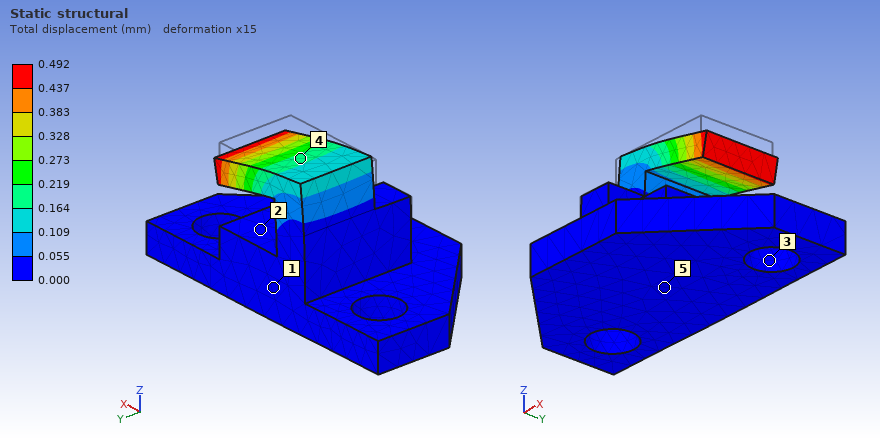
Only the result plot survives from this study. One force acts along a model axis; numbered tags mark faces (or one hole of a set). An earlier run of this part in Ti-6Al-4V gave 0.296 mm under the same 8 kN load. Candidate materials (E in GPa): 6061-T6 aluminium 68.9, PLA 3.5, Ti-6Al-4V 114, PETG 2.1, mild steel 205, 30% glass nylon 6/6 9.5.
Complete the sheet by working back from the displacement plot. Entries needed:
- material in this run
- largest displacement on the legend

6061-T6 aluminium
0.492 mm
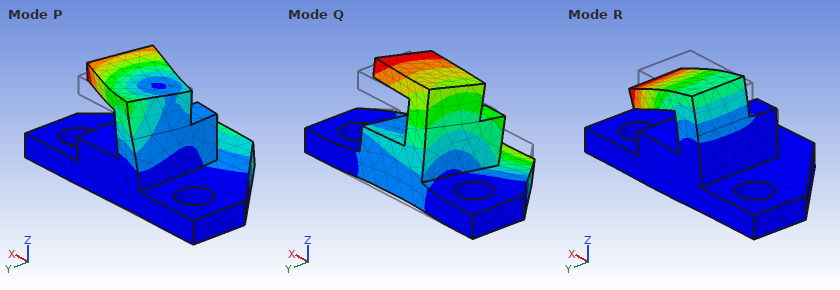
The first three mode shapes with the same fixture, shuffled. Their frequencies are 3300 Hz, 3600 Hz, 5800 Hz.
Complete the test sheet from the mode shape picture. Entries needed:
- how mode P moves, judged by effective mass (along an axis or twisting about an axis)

along Z
